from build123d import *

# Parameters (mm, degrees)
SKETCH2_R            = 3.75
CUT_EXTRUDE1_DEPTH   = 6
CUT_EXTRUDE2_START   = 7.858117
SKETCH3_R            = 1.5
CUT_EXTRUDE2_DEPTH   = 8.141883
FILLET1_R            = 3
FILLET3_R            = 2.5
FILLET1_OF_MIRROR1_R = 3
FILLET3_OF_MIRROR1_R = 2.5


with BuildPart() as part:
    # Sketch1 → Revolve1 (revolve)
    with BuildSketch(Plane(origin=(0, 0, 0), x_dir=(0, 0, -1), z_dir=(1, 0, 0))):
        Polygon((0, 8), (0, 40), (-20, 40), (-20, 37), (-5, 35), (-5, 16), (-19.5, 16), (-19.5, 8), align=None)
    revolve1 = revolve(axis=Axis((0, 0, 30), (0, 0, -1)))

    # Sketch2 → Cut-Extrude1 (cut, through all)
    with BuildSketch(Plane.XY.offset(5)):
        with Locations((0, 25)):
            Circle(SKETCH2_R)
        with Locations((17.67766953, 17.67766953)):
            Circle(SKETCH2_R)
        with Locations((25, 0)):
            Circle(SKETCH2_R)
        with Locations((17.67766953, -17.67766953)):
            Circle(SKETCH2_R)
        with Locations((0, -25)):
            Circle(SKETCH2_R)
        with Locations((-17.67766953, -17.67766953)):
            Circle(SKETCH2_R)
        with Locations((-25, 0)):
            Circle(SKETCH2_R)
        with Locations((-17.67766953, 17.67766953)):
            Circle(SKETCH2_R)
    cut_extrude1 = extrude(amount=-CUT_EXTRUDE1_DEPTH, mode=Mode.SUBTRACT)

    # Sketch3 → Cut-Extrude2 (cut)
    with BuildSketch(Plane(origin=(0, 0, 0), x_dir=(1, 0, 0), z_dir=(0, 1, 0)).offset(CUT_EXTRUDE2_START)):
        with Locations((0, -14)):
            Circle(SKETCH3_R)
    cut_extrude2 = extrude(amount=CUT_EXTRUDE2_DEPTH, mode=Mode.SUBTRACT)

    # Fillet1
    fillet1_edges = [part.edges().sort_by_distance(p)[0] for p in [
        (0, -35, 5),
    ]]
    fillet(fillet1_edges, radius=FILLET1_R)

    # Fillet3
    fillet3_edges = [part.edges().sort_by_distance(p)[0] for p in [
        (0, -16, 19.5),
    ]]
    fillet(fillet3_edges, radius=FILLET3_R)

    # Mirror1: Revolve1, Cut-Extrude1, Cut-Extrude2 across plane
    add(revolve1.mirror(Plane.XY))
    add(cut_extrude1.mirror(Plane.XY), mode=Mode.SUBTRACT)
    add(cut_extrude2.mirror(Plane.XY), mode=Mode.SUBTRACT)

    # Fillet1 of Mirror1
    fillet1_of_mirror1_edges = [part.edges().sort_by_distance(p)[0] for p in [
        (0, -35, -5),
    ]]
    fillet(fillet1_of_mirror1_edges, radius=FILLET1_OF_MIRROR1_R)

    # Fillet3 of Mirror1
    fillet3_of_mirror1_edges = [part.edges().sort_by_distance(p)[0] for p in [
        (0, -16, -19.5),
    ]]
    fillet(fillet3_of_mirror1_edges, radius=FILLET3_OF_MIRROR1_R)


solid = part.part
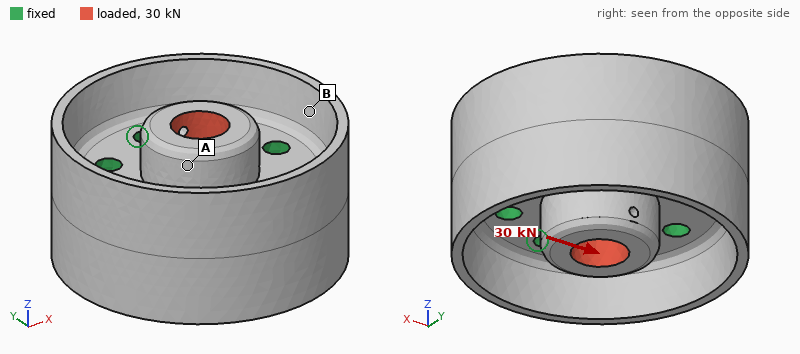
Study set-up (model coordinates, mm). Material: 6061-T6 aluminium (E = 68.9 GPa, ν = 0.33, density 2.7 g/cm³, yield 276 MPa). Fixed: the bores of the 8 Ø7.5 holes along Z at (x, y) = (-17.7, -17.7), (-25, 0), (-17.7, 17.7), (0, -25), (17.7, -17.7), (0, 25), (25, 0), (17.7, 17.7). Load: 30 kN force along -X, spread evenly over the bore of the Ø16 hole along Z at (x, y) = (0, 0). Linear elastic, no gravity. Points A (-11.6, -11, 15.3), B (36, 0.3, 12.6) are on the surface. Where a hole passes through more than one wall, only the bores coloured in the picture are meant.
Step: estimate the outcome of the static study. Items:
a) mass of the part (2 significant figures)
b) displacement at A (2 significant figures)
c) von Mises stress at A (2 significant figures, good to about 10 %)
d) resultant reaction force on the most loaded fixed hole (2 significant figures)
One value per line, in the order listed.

250 g
14 µm
13 MPa
6.2 kN
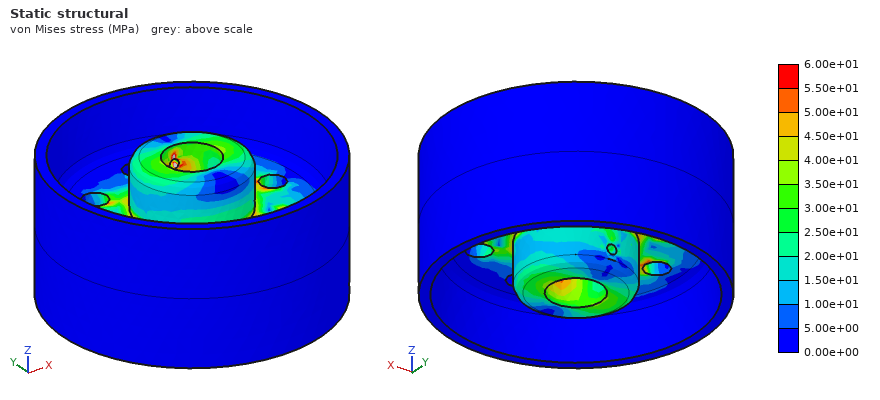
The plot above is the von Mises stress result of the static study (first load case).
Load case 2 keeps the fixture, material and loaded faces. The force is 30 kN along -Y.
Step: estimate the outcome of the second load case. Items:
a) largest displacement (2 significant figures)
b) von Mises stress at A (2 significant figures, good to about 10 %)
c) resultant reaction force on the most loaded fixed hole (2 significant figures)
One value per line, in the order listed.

20 µm
12 MPa
6.2 kN
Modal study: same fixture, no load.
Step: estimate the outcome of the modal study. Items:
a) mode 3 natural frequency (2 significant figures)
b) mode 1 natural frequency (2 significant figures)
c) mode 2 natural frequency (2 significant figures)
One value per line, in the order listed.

14 kHz
13 kHz
13 kHz
